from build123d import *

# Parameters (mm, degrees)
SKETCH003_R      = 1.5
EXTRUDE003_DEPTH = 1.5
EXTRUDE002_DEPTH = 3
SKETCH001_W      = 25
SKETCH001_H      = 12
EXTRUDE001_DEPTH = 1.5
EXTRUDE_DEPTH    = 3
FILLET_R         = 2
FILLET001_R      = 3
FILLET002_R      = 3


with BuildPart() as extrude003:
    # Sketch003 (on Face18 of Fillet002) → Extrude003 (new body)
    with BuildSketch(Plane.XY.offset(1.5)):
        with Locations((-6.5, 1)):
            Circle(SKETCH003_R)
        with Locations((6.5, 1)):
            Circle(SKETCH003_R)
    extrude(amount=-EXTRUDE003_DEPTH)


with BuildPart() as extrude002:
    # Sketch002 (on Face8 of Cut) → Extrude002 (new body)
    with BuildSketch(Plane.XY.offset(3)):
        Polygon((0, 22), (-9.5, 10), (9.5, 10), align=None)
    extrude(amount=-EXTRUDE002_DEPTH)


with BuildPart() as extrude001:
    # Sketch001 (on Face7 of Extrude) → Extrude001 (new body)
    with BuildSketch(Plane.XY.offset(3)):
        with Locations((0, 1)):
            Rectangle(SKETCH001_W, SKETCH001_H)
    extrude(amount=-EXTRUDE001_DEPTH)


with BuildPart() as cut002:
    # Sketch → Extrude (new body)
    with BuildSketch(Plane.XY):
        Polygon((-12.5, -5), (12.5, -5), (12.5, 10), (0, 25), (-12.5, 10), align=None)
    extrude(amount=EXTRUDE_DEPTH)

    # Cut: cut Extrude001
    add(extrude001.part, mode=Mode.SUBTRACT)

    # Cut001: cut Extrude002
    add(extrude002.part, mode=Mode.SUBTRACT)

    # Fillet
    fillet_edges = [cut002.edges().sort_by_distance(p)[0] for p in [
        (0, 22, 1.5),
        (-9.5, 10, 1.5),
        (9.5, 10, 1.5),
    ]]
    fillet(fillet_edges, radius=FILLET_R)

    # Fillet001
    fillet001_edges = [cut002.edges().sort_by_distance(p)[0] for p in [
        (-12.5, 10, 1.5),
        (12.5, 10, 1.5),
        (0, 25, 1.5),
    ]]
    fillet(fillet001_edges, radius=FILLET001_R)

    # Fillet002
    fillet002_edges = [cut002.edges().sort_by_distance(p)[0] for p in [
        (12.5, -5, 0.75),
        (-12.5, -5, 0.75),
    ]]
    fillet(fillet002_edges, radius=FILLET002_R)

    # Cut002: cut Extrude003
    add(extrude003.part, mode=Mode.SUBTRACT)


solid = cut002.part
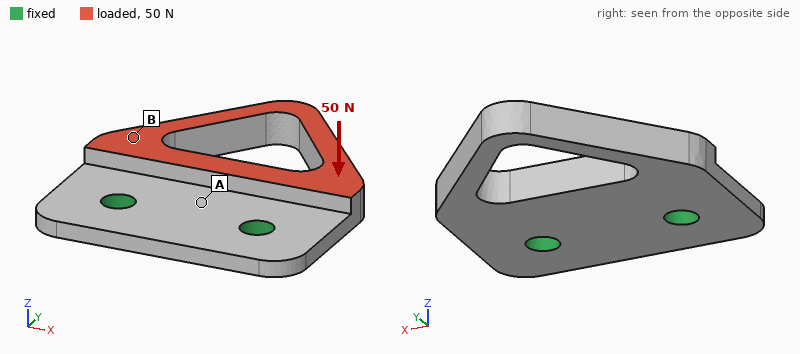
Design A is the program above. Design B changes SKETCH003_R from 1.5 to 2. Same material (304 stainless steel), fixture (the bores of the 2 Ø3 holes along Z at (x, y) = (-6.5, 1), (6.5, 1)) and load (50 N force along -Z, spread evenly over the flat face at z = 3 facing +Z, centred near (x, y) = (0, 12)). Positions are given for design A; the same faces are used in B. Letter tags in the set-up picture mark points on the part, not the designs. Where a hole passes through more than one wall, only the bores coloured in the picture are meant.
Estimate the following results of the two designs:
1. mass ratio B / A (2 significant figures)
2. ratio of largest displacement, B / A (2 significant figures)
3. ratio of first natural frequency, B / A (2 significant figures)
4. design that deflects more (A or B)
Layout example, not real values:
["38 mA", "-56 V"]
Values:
["0.98", "0.86", "1.1", "A"]
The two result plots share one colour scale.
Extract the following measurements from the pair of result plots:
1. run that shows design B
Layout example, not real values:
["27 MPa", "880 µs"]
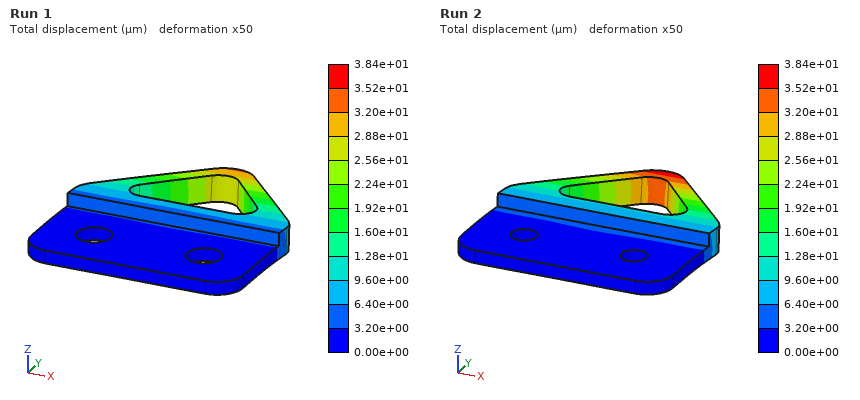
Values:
["Run 1"]
